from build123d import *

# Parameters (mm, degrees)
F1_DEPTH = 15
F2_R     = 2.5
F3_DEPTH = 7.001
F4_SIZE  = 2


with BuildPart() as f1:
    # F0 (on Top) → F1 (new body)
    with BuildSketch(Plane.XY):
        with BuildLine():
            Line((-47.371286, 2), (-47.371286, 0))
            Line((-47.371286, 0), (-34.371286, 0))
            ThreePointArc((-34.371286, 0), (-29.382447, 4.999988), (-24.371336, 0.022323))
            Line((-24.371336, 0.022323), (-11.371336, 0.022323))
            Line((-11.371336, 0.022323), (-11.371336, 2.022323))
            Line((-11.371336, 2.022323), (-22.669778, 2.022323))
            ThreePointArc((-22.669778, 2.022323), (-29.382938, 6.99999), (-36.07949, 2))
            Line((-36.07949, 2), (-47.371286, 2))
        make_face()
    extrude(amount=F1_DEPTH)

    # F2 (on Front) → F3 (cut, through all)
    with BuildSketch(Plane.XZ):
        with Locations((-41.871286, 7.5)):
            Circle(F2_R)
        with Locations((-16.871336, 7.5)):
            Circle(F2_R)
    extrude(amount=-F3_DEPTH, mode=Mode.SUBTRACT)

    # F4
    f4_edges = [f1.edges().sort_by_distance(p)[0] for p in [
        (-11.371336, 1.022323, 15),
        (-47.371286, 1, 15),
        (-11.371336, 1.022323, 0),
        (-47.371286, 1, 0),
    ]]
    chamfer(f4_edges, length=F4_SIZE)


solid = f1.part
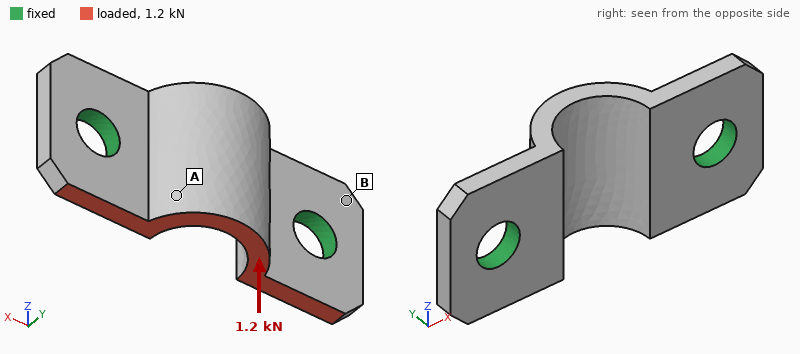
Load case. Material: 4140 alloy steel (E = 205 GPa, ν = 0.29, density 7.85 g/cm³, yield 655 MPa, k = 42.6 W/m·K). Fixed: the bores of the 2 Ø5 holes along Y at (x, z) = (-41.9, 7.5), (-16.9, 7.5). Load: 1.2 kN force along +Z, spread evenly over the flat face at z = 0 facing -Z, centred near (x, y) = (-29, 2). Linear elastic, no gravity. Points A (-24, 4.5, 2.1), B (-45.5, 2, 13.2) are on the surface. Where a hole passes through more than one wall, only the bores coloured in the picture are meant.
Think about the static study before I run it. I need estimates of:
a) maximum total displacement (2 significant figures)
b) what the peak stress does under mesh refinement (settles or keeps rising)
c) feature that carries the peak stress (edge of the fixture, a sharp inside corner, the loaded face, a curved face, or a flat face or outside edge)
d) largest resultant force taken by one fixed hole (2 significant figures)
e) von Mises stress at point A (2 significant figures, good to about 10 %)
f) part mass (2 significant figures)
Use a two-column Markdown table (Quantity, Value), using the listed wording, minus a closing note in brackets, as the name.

| Quantity | Value |
|---|---|
| maximum total displacement | 12 µm |
| what the peak stress does under mesh refinement | keeps rising |
| feature that carries the peak stress | edge of the fixture |
| largest resultant force taken by one fixed hole | 600 N |
| von Mises stress at point A | 29 MPa |
| part mass | 8.9 g |
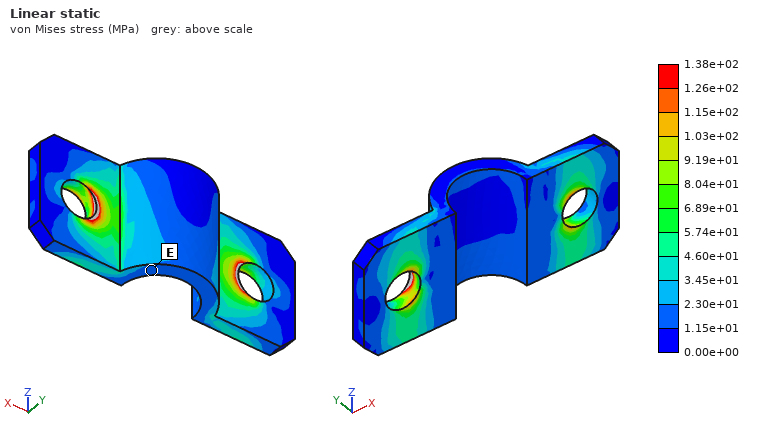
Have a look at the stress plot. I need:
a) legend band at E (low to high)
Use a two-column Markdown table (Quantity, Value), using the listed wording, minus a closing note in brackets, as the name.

| Quantity | Value |
|---|---|
| legend band at E | 1.15e+01 to 2.30e+01 MPa |
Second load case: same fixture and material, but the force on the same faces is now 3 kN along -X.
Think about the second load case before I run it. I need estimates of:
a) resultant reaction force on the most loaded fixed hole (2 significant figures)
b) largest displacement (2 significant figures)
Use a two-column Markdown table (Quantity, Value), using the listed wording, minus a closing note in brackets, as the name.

| Quantity | Value |
|---|---|
| resultant reaction force on the most loaded fixed hole | 1.6 kN |
| largest displacement | 18 µm |
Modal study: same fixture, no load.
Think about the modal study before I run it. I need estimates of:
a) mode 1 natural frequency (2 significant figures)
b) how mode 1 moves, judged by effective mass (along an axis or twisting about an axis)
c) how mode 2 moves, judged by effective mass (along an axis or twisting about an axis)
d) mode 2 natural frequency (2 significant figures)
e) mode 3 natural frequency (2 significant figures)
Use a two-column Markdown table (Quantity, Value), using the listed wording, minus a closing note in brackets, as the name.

| Quantity | Value |
|---|---|
| mode 1 natural frequency | 17 kHz |
| how mode 1 moves, judged by effective mass | along Z |
| how mode 2 moves, judged by effective mass | along Y |
| mode 2 natural frequency | 28 kHz |
| mode 3 natural frequency | 37 kHz |
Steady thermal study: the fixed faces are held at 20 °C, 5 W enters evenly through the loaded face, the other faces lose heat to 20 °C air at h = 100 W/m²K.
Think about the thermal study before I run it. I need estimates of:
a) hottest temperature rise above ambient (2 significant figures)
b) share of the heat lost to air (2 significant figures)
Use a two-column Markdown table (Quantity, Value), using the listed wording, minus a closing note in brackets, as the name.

| Quantity | Value |
|---|---|
| hottest temperature rise above ambient | 17 K |
| share of the heat lost to air | 14 % |
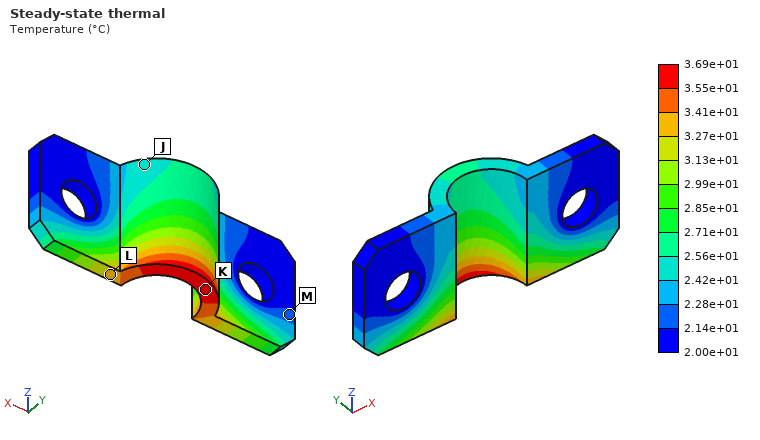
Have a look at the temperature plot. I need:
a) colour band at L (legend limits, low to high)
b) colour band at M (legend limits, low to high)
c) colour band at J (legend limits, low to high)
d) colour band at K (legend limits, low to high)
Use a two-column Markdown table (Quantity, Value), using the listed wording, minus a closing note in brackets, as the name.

| Quantity | Value |
|---|---|
| colour band at L | 3.27e+01 to 3.41e+01 °C |
| colour band at M | 2.14e+01 to 2.28e+01 °C |
| colour band at J | 2.42e+01 to 2.56e+01 °C |
| colour band at K | 3.55e+01 to 3.69e+01 °C |
